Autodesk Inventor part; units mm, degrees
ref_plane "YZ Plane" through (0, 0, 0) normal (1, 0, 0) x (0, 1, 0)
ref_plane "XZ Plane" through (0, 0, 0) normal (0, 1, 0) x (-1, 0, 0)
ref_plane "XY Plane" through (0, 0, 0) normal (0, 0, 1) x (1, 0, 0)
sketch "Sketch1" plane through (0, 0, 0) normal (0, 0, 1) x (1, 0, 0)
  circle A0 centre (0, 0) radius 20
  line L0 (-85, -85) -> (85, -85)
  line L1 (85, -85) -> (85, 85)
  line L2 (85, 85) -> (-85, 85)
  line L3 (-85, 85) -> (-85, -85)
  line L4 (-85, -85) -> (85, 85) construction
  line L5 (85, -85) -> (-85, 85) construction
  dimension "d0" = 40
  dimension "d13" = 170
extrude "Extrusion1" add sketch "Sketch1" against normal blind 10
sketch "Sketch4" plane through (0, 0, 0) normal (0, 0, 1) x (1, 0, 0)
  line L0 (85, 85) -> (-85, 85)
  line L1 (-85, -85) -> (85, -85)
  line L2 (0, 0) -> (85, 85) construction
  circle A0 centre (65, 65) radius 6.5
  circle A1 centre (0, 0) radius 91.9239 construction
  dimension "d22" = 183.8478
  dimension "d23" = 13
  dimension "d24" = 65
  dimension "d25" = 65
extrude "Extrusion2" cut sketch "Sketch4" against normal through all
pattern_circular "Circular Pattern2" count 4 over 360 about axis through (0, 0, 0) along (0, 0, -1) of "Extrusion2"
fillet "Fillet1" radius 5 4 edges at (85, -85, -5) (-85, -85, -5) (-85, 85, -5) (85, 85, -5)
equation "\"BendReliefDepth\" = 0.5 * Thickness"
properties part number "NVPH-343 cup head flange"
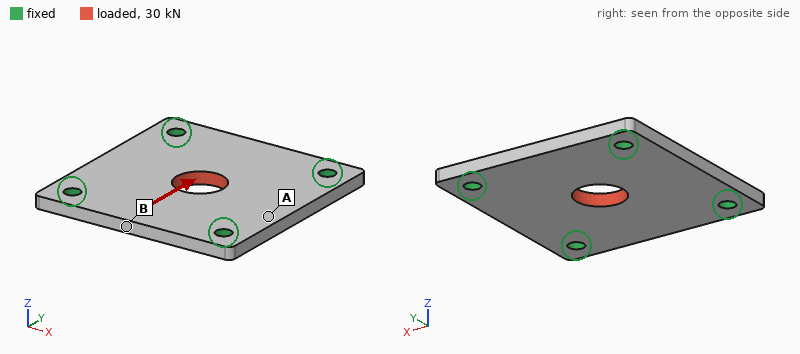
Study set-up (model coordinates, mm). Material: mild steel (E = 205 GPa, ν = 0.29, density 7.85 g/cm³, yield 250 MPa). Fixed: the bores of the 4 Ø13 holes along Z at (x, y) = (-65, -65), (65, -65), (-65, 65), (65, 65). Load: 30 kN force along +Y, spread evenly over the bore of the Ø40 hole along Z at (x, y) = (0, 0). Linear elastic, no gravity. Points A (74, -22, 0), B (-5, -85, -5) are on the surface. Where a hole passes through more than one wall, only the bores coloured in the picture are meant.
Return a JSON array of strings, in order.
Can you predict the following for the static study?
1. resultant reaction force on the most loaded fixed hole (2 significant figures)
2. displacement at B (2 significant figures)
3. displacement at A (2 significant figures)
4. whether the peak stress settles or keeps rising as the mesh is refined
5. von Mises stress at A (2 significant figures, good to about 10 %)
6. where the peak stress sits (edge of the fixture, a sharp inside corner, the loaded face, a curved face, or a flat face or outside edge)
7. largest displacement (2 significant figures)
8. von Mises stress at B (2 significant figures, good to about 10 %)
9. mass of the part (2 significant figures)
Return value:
["8.3 kN", "6.6 µm", "1.9 µm", "keeps rising", "5.6 MPa", "edge of the fixture", "9.8 µm", "15 MPa", "2.1 kg"]
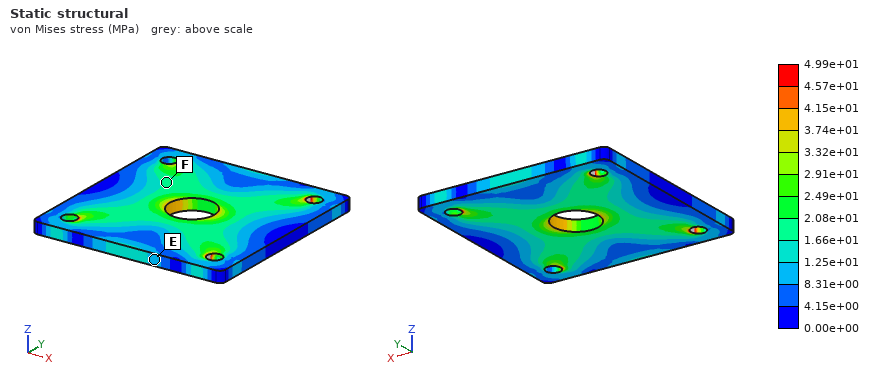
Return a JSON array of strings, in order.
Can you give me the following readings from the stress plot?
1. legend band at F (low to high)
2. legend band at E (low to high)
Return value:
["1.66e+01 to 2.08e+01 MPa", "8.31e+00 to 1.25e+01 MPa"]
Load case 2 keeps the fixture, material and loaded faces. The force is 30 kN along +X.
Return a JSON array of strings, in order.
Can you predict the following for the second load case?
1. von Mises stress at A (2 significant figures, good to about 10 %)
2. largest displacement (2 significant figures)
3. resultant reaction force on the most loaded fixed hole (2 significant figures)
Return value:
["7.6 MPa", "9.8 µm", "8.3 kN"]
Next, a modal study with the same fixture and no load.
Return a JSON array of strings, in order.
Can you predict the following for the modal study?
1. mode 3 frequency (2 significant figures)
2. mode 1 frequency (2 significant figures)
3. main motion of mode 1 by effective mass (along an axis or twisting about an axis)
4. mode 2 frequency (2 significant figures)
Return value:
["3500 Hz", "2300 Hz", "along Z", "3500 Hz"]
